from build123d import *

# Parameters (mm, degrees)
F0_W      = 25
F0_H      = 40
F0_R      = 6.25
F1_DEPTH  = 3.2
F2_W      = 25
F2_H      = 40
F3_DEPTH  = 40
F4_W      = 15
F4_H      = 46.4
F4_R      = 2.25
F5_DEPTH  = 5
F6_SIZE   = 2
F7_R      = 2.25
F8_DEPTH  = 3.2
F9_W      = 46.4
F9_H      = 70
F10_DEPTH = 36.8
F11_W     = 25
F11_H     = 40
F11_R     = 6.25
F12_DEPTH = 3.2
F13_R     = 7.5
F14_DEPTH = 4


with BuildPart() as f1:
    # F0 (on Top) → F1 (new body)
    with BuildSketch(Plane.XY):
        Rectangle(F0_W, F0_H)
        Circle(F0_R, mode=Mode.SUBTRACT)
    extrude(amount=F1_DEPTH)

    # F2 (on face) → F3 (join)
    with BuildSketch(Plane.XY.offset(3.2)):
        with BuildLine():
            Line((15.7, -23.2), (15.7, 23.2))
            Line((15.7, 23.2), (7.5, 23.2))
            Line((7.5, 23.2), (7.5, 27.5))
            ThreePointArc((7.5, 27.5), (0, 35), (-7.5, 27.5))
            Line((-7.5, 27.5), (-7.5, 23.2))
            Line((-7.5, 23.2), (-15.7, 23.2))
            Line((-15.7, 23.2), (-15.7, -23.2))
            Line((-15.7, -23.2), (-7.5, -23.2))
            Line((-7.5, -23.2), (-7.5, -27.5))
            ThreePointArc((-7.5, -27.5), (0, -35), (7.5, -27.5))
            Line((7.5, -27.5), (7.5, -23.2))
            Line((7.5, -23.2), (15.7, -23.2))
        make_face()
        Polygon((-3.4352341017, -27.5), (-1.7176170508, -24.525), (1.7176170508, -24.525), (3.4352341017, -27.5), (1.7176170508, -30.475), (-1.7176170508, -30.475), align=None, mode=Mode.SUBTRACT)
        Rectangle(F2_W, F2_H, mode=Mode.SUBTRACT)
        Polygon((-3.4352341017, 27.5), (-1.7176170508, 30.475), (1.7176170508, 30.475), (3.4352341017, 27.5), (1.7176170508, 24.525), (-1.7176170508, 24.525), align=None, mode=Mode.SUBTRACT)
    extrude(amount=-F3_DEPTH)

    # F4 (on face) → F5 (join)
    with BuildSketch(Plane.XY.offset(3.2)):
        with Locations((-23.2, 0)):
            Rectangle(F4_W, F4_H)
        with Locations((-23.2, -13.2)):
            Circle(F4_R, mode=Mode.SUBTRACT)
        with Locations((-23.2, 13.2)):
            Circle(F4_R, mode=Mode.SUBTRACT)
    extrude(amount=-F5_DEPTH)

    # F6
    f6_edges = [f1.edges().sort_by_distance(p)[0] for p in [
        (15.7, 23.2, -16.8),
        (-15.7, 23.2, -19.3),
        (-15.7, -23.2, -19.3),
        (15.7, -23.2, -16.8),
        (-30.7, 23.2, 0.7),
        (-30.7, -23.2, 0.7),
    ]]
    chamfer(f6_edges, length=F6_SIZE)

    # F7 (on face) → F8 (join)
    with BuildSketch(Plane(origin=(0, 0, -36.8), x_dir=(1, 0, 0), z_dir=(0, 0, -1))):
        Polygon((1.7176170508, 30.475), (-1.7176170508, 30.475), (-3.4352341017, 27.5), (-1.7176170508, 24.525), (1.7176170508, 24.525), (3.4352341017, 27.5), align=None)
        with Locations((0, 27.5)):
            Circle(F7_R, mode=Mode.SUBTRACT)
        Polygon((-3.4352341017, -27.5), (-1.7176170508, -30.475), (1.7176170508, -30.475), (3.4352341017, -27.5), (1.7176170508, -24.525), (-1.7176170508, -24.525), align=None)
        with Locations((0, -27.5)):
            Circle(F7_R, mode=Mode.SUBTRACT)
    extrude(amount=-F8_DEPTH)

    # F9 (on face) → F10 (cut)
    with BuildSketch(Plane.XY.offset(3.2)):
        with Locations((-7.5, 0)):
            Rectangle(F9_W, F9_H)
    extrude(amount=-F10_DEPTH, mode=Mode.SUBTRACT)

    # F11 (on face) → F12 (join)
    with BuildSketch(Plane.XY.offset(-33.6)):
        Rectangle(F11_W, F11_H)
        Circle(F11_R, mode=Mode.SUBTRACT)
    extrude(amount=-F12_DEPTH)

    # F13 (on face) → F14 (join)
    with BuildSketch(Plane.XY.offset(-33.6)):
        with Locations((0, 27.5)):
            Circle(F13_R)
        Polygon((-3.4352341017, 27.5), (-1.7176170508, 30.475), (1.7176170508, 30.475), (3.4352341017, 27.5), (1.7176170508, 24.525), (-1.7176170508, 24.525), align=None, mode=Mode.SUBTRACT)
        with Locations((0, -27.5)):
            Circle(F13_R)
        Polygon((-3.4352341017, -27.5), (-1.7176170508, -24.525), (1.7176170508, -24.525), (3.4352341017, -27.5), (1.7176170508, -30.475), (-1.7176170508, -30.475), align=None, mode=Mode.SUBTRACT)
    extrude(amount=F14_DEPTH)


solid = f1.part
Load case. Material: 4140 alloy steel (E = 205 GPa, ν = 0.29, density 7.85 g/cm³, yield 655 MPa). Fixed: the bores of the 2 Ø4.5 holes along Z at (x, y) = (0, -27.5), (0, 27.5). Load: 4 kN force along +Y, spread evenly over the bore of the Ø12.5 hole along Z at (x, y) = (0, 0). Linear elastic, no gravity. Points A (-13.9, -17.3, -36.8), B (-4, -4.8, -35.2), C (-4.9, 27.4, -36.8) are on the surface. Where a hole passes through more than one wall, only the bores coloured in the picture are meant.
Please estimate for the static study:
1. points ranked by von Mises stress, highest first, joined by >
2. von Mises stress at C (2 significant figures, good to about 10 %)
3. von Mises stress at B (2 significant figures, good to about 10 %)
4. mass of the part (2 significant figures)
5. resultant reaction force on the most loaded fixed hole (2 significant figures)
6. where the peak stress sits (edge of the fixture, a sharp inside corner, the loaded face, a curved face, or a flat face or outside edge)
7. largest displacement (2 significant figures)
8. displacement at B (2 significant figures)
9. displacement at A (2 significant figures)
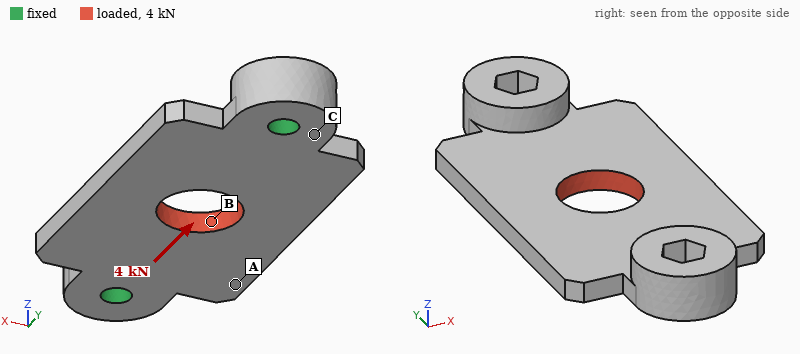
B > C > A
24 MPa
43 MPa
49 g
2.0 kN
edge of the fixture
4.6 µm
4.2 µm
3.0 µm
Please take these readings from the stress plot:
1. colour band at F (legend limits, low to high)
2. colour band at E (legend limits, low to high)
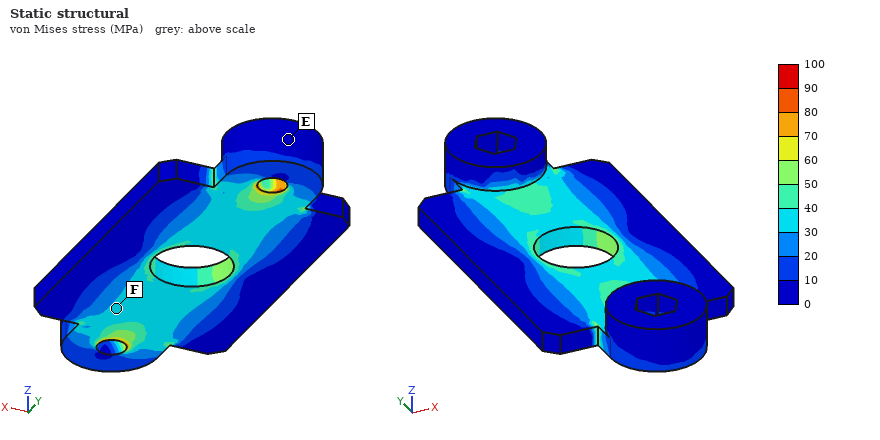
30 to 40 MPa
0 to 10 MPa
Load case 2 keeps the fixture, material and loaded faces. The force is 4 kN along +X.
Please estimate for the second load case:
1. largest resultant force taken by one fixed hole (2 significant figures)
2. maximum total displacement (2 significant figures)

2.0 kN
15 µm
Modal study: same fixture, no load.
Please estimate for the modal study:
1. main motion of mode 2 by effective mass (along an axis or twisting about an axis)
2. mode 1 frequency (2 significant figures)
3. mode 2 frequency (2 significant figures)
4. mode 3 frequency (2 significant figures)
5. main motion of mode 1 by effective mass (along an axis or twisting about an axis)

twisting about Y
5400 Hz
5900 Hz
12 kHz
along Z
